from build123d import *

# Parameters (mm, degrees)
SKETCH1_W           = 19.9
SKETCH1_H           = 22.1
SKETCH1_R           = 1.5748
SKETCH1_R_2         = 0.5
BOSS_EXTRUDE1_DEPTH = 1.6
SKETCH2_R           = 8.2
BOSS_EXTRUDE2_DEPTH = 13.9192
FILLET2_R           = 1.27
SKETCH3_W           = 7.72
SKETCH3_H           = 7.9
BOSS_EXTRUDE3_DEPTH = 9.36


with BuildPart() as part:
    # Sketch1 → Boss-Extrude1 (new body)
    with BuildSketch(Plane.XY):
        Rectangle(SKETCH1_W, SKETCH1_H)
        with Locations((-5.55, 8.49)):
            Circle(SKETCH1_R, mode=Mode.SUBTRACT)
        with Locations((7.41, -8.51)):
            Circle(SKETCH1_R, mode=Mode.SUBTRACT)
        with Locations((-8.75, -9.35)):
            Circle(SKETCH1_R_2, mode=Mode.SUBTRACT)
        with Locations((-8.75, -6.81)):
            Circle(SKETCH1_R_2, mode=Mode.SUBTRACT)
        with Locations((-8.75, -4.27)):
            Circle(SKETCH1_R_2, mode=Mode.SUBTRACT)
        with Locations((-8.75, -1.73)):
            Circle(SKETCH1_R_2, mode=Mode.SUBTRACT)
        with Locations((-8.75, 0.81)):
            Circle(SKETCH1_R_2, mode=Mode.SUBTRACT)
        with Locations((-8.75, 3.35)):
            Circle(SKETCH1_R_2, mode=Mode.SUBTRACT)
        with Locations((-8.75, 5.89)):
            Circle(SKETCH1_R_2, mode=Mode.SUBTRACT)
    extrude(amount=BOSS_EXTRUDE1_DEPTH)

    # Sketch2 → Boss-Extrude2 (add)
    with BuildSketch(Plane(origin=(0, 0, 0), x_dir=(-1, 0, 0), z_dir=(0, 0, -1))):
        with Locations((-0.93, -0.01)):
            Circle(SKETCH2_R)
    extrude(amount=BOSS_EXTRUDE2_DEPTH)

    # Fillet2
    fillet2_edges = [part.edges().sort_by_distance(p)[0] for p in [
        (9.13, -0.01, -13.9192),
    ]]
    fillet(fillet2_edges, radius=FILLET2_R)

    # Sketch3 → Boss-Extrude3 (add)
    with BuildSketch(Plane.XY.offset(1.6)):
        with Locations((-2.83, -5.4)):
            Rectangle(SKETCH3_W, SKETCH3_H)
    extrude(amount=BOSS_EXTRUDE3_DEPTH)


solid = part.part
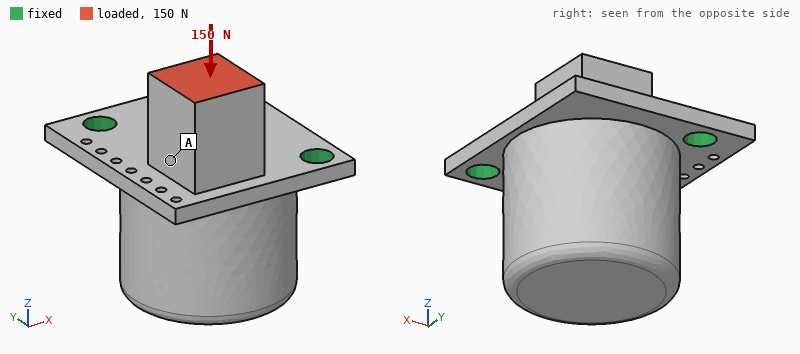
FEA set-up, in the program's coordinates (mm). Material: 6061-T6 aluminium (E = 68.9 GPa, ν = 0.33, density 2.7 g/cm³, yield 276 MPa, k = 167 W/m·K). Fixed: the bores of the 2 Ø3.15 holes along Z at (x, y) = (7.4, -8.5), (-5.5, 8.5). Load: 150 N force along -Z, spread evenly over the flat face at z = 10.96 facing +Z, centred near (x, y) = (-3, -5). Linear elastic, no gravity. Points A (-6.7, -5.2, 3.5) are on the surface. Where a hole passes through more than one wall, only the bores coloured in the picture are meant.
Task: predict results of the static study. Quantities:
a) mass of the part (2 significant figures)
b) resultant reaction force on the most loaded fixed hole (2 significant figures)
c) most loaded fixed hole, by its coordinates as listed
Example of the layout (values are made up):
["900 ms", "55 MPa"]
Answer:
["11 g", "98 N", "(7.4, -8.5)"]
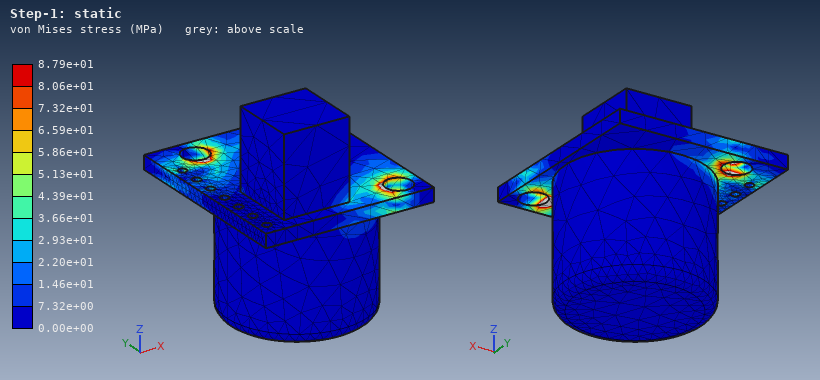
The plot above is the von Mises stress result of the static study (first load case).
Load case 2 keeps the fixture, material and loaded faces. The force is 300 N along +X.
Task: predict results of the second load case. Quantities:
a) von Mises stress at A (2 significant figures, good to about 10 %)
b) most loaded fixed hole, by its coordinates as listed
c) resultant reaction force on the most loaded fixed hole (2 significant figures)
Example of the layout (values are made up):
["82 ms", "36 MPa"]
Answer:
["29 MPa", "(7.4, -8.5)", "260 N"]
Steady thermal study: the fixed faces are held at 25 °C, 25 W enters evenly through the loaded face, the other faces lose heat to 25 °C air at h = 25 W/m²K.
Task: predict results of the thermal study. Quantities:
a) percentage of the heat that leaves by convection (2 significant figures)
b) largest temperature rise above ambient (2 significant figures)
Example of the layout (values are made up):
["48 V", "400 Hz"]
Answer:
["3.9 %", "50 K"]
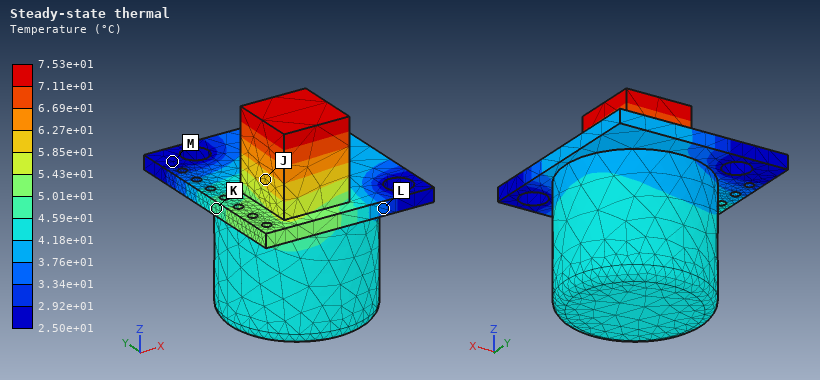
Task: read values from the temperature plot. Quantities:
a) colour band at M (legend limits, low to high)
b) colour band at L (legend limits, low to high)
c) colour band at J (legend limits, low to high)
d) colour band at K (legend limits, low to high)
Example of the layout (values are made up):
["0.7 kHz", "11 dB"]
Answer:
["2.50e+01 to 2.92e+01 °C", "3.34e+01 to 3.76e+01 °C", "5.85e+01 to 6.27e+01 °C", "4.59e+01 to 5.01e+01 °C"]
